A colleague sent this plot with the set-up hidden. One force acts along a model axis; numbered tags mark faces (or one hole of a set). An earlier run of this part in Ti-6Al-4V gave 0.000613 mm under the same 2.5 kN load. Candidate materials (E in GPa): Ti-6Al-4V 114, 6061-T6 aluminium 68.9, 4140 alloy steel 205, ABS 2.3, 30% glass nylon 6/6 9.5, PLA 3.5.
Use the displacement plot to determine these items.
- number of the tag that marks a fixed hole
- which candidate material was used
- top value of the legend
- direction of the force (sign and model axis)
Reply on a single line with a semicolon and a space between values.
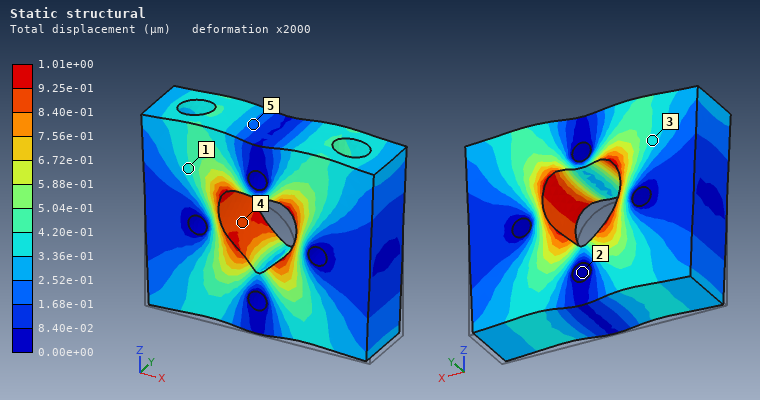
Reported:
2; 6061-T6 aluminium; 1.01e+00 µm; +Z
